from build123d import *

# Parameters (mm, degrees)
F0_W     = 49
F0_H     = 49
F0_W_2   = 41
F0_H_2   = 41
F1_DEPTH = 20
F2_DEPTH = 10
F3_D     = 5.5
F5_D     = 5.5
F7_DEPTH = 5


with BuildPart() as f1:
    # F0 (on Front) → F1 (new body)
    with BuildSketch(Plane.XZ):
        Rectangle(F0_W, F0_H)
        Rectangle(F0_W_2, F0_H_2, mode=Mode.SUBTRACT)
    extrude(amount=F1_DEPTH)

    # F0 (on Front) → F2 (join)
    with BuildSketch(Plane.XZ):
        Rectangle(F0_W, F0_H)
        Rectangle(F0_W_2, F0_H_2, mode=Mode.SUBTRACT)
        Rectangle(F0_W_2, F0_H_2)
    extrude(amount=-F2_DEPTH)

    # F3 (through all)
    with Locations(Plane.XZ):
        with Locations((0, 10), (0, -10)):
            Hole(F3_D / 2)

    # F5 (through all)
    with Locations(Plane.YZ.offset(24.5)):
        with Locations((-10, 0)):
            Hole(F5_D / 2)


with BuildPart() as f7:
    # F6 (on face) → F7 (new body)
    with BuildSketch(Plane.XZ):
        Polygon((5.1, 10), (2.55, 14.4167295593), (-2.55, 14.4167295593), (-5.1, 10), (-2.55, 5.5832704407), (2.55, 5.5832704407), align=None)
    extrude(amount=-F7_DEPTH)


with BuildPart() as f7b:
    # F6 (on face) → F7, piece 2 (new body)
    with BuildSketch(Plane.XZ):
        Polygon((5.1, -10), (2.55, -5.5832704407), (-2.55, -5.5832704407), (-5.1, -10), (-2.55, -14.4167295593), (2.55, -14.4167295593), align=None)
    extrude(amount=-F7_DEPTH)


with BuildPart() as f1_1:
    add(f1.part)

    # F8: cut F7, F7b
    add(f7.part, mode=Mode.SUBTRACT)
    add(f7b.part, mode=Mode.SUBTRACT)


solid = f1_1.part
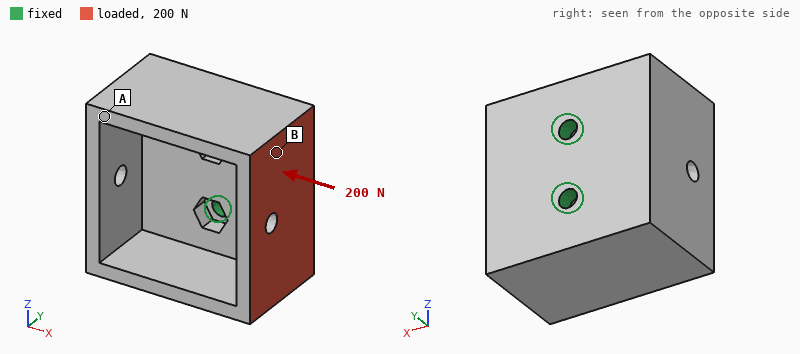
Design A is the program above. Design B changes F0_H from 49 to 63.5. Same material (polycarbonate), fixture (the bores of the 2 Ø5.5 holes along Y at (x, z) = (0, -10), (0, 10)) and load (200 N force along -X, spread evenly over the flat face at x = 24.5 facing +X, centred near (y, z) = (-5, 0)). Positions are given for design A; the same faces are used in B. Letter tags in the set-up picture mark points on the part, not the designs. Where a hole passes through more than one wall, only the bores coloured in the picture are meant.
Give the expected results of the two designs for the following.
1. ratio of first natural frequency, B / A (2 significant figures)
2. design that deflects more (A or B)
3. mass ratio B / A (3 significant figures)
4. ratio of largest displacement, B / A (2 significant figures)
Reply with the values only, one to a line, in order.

0.78
A
1.57
0.84
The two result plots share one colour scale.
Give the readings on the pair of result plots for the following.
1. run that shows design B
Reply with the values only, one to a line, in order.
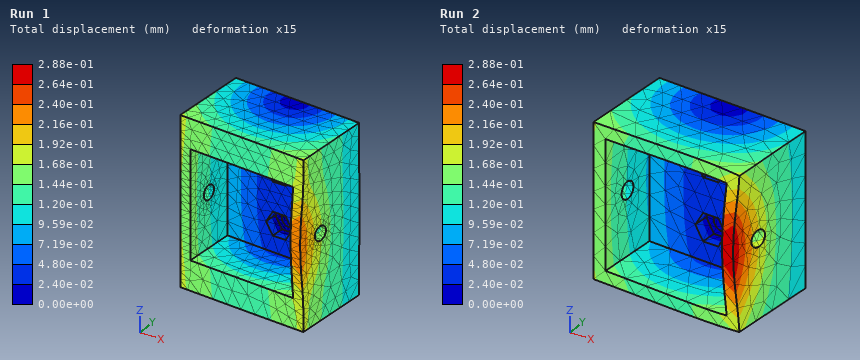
Run 1
